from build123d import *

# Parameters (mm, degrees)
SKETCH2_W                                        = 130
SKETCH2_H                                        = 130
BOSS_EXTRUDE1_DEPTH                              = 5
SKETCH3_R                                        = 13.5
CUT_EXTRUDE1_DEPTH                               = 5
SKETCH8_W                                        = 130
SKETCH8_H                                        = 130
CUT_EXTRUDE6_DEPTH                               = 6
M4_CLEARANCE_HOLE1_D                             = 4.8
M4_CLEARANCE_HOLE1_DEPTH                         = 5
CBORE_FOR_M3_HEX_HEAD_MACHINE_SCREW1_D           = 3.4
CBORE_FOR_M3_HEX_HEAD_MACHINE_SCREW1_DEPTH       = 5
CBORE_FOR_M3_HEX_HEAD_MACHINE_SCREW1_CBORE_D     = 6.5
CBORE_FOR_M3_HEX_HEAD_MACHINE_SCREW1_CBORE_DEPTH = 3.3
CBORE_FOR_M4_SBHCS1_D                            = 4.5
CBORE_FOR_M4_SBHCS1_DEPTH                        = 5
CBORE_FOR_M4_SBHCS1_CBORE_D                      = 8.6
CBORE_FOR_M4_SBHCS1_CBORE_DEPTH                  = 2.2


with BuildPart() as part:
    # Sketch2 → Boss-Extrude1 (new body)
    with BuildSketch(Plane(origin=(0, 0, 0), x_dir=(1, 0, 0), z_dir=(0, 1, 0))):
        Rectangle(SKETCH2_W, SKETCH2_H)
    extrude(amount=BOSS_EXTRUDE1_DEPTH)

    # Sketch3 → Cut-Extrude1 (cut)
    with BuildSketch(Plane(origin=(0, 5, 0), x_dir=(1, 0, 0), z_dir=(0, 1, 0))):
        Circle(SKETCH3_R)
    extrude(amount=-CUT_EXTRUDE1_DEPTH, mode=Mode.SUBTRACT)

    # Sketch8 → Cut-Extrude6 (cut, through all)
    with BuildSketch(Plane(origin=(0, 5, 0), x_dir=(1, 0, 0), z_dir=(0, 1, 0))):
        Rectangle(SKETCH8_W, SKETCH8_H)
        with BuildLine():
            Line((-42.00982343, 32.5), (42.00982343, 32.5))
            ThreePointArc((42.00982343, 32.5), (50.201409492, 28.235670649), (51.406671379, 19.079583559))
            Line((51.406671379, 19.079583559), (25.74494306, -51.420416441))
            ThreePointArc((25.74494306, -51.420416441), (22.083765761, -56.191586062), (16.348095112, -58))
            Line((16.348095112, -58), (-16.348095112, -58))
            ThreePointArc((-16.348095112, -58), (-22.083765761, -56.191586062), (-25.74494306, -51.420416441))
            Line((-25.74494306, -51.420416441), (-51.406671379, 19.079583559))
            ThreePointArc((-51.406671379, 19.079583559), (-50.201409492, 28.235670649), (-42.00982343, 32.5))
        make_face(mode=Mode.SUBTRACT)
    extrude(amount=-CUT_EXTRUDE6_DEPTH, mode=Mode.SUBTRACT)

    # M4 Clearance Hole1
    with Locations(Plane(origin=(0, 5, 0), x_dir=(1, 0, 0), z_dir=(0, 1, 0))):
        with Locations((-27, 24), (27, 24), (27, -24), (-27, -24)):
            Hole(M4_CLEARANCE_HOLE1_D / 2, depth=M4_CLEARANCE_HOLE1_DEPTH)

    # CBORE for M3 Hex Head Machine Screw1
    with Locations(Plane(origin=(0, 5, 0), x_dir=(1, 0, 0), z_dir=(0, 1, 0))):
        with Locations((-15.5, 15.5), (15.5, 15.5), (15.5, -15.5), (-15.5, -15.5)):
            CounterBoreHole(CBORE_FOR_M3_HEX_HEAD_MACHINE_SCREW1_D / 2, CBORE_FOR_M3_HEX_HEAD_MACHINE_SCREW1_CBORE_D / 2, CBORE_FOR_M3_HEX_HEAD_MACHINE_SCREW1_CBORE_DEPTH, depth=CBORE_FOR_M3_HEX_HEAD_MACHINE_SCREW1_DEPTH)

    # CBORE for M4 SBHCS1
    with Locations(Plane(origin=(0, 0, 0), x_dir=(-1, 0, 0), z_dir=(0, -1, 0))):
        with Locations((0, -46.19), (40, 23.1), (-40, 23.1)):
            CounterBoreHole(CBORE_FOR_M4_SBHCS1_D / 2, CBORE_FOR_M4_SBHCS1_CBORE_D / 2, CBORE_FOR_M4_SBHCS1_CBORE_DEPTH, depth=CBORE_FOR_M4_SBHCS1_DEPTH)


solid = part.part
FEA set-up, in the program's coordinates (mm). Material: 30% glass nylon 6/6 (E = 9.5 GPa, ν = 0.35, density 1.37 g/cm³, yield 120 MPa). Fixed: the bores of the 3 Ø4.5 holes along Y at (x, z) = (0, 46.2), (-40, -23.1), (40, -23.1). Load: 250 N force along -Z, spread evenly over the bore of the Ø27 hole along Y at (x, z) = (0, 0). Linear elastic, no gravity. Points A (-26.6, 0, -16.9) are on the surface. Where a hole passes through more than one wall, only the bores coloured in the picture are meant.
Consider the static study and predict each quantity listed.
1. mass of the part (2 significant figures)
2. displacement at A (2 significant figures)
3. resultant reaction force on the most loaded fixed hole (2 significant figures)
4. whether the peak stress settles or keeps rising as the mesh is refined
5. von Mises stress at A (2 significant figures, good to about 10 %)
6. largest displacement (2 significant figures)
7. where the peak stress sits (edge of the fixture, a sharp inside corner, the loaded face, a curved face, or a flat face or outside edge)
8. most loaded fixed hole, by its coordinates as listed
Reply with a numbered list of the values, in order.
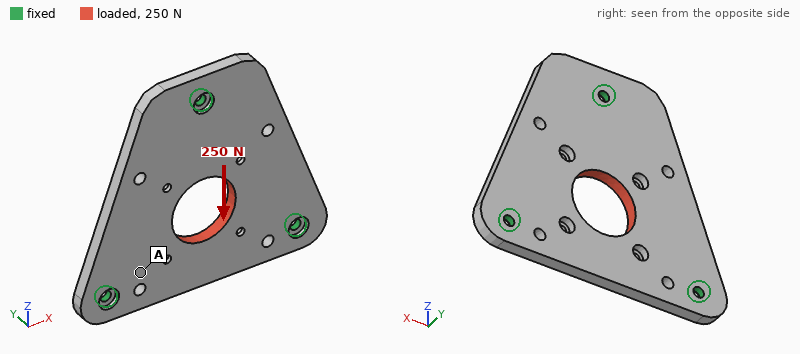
1. 43 g
2. 4.0 µm
3. 110 N
4. keeps rising
5. 0.54 MPa
6. 8.8 µm
7. edge of the fixture
8. (0, 46.2)
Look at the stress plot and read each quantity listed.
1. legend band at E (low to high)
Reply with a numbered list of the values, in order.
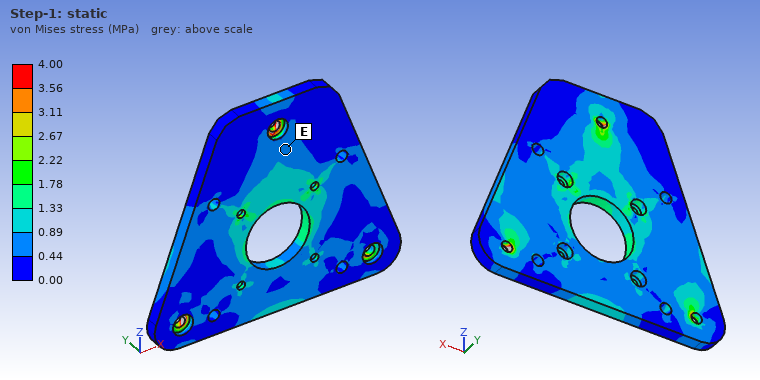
1. 0.44 to 0.89 MPa
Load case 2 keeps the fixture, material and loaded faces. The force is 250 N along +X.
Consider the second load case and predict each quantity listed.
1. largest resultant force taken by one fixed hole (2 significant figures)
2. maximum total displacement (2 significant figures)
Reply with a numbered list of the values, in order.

1. 89 N
2. 6.8 µm
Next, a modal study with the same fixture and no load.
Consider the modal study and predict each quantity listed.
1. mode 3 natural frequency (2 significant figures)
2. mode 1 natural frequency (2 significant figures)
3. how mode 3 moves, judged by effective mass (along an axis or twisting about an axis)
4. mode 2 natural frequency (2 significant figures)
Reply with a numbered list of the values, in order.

1. 1900 Hz
2. 1500 Hz
3. twisting about X
4. 1500 Hz
